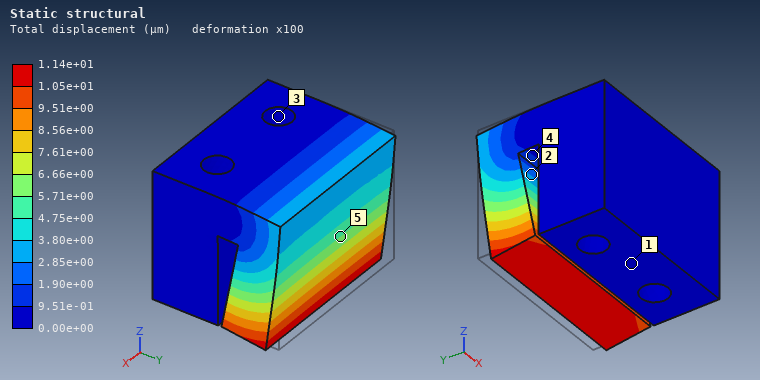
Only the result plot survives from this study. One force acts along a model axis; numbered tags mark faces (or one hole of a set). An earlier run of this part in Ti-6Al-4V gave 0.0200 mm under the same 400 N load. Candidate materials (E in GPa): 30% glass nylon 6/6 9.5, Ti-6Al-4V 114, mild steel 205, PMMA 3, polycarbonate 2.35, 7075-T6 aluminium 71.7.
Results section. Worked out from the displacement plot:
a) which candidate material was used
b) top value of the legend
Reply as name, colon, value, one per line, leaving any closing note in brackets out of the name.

which candidate material was used: mild steel
top value of the legend: 1.14e+01 µm
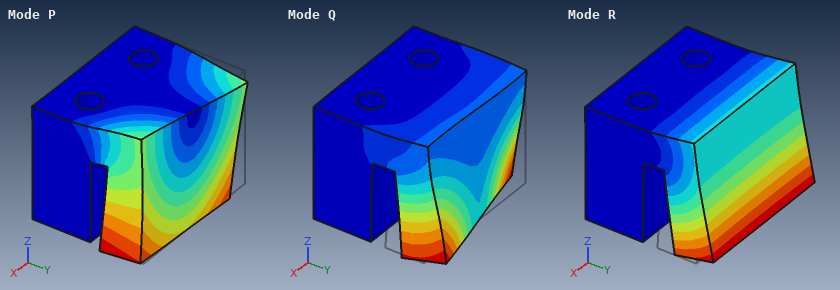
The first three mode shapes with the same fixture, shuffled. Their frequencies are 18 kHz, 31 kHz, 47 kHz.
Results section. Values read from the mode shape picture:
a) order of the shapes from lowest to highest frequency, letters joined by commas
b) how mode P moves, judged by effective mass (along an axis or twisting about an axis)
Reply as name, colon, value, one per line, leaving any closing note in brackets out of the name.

order of the shapes from lowest to highest frequency, letters joined by commas: R, P, Q
how mode P moves, judged by effective mass: along X
